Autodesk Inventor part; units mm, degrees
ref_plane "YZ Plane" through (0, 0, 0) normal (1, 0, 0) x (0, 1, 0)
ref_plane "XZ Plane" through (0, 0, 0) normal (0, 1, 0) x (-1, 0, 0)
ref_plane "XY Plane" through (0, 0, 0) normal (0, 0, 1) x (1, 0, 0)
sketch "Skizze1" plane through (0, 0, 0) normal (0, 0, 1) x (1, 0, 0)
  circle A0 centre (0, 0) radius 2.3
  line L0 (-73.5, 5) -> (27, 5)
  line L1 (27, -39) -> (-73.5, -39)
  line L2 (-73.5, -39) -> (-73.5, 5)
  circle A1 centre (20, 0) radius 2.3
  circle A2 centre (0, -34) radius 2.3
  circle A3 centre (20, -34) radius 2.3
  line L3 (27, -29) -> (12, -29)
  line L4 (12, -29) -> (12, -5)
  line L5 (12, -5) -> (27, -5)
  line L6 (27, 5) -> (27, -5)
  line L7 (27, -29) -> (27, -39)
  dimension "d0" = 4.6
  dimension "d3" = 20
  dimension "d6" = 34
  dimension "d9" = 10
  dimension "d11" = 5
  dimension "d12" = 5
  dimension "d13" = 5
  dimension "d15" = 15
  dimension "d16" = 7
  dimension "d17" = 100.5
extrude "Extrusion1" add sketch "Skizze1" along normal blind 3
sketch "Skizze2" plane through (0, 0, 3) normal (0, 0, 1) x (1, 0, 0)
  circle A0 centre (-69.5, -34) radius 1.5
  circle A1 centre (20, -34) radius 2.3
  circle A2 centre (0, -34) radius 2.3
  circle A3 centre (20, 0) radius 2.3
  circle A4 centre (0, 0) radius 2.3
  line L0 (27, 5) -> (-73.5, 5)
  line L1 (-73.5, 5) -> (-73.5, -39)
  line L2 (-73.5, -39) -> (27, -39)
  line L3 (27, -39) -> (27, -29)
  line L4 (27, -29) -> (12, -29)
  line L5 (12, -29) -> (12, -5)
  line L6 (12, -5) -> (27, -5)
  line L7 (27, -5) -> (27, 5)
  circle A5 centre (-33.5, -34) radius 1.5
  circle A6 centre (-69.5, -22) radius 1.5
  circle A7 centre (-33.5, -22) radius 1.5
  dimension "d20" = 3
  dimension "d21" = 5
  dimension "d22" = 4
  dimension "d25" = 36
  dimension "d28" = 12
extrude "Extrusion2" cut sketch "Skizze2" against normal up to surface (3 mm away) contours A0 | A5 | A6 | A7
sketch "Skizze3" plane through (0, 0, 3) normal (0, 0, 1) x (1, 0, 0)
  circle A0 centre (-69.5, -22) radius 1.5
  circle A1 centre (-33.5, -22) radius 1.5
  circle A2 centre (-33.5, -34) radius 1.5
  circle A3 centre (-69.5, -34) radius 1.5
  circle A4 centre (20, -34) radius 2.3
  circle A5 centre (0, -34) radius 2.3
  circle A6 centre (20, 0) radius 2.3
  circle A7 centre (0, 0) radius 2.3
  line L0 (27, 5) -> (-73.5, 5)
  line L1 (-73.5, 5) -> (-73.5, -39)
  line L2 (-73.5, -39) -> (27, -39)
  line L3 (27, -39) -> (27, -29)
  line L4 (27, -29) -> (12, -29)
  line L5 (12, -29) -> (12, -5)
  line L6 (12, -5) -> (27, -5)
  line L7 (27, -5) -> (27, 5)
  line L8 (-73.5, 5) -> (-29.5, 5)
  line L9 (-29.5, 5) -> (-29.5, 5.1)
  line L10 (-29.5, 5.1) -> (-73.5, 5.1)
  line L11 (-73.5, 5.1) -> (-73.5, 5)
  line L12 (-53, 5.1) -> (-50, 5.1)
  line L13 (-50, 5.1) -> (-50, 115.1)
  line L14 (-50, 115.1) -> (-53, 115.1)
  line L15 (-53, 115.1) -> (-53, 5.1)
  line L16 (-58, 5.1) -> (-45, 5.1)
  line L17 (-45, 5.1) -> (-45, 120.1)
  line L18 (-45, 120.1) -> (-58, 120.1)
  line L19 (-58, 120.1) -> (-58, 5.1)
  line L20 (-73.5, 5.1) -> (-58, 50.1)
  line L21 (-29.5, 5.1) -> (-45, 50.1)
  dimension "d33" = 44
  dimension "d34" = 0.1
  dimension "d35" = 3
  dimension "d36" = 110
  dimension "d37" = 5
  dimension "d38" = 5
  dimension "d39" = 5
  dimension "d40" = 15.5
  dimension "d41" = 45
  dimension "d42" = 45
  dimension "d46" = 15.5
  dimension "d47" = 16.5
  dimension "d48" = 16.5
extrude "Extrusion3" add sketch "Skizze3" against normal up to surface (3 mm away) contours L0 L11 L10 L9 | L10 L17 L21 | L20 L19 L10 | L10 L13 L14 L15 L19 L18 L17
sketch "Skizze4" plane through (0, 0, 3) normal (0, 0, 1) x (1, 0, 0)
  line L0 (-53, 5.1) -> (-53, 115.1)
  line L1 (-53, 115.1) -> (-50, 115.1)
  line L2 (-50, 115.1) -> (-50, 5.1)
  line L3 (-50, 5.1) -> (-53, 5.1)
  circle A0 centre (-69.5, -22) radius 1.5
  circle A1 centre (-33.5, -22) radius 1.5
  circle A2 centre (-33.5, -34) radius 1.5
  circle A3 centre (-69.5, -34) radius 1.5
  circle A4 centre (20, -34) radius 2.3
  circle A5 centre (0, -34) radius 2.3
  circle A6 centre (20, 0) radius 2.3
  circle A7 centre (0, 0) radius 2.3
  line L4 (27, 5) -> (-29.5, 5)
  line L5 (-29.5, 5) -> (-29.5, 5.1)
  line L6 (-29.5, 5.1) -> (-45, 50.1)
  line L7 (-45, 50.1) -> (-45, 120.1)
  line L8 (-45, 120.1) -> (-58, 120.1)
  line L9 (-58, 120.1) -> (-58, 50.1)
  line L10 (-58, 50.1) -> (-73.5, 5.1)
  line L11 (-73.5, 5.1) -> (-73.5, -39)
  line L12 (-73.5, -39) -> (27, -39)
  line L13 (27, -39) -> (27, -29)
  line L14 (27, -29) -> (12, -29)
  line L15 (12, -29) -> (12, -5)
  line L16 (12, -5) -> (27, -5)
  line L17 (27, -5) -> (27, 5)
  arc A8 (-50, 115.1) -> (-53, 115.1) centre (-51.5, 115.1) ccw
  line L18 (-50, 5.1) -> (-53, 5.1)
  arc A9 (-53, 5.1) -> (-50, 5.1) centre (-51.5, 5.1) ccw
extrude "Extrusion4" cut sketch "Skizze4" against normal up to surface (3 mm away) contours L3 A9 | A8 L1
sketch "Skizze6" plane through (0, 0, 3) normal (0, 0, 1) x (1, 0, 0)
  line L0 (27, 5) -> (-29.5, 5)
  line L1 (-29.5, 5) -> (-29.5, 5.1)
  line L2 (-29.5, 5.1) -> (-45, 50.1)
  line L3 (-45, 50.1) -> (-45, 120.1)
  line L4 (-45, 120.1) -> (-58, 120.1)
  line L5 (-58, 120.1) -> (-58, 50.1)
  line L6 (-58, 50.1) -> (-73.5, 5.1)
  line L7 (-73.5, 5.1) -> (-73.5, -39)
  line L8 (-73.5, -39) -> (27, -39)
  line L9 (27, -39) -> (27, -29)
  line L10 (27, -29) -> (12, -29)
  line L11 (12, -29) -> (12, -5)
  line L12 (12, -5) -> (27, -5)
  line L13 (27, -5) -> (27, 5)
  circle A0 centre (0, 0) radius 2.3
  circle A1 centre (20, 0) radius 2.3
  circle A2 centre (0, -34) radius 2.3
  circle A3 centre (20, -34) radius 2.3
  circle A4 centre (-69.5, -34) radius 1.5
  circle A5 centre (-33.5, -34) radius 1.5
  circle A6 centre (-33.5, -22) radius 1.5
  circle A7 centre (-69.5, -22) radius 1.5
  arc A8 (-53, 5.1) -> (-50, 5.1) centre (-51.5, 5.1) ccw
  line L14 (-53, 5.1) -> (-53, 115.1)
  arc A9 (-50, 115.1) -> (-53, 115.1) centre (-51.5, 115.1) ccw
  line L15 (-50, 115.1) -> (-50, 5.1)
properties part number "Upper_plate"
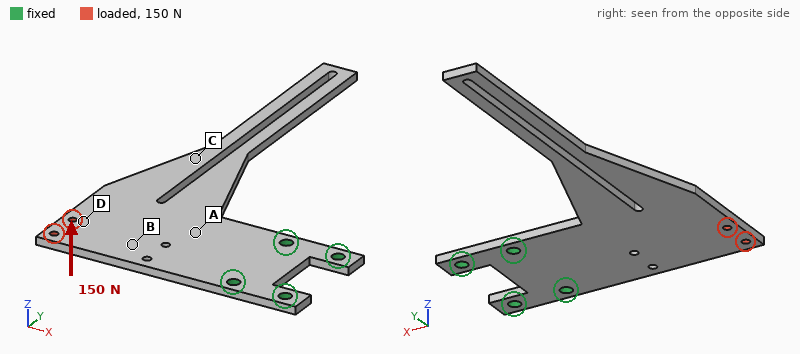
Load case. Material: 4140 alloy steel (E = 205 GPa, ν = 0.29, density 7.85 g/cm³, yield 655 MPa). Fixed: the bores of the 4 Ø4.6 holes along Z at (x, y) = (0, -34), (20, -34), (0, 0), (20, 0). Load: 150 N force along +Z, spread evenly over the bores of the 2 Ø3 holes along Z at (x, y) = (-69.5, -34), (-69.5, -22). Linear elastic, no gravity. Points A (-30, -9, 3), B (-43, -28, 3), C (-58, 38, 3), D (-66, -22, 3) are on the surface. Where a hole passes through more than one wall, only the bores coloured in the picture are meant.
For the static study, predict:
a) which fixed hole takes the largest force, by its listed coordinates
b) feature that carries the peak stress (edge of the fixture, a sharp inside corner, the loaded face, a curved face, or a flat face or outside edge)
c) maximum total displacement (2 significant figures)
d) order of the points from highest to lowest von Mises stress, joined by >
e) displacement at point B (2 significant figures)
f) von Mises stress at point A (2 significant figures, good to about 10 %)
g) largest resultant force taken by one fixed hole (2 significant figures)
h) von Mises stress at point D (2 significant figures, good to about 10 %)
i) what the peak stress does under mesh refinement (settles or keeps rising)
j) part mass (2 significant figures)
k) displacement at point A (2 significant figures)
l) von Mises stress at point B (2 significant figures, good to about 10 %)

(0, -34)
edge of the fixture
0.96 mm
A > B > D > C
0.40 mm
88 MPa
190 N
34 MPa
keeps rising
140 g
0.19 mm
64 MPa
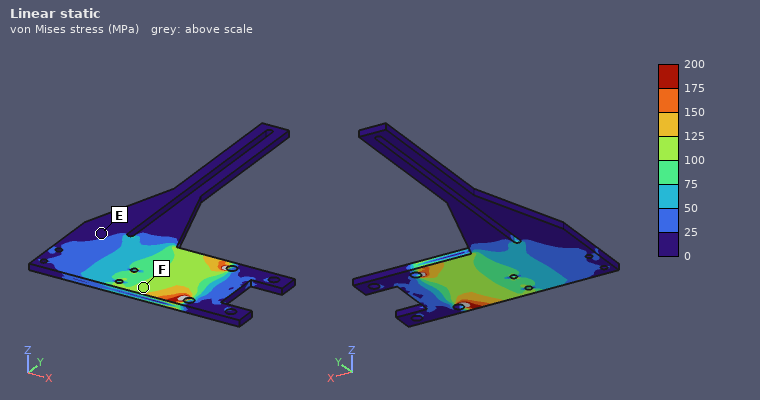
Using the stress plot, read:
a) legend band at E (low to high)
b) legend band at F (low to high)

0 to 25 MPa
100 to 125 MPa
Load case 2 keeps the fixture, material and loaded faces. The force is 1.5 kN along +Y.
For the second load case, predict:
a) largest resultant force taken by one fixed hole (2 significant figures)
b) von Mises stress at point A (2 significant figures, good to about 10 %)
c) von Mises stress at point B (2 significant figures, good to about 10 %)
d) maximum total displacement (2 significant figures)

2.9 kN
36 MPa
28 MPa
0.12 mm
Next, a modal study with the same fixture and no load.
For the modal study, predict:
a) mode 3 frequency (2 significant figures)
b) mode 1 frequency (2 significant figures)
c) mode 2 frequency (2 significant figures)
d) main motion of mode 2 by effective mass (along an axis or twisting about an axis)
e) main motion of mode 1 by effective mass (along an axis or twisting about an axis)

860 Hz
190 Hz
390 Hz
along Z
along Z
